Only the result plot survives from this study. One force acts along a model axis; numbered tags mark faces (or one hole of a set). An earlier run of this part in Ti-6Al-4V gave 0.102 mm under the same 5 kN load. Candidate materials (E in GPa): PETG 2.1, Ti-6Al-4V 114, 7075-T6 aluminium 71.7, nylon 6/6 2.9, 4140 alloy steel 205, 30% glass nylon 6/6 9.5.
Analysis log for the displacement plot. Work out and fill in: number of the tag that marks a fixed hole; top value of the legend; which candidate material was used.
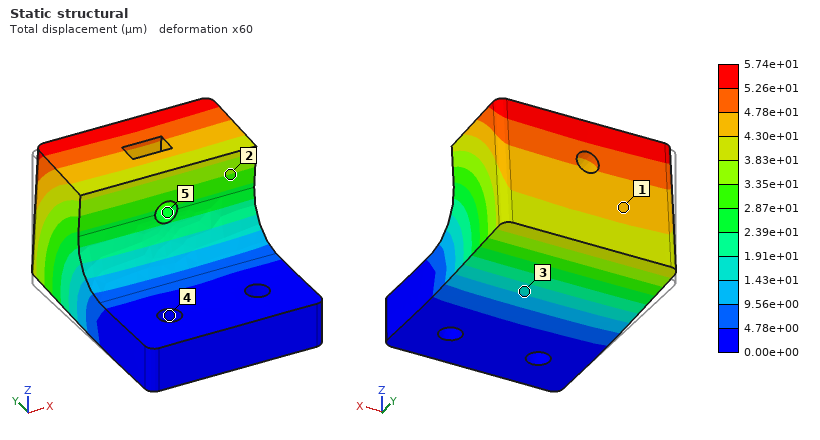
4
5.74e+01 µm
4140 alloy steel
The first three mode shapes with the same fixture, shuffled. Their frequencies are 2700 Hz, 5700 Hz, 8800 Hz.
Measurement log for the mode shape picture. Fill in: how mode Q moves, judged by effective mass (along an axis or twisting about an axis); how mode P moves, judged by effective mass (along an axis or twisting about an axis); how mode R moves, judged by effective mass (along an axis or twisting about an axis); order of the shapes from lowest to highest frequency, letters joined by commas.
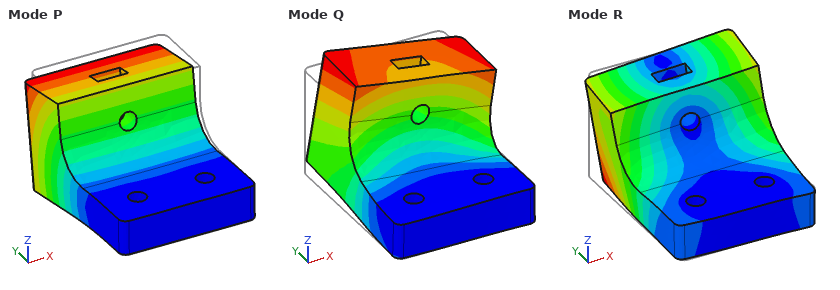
along X
along Z
along X
P, Q, R
